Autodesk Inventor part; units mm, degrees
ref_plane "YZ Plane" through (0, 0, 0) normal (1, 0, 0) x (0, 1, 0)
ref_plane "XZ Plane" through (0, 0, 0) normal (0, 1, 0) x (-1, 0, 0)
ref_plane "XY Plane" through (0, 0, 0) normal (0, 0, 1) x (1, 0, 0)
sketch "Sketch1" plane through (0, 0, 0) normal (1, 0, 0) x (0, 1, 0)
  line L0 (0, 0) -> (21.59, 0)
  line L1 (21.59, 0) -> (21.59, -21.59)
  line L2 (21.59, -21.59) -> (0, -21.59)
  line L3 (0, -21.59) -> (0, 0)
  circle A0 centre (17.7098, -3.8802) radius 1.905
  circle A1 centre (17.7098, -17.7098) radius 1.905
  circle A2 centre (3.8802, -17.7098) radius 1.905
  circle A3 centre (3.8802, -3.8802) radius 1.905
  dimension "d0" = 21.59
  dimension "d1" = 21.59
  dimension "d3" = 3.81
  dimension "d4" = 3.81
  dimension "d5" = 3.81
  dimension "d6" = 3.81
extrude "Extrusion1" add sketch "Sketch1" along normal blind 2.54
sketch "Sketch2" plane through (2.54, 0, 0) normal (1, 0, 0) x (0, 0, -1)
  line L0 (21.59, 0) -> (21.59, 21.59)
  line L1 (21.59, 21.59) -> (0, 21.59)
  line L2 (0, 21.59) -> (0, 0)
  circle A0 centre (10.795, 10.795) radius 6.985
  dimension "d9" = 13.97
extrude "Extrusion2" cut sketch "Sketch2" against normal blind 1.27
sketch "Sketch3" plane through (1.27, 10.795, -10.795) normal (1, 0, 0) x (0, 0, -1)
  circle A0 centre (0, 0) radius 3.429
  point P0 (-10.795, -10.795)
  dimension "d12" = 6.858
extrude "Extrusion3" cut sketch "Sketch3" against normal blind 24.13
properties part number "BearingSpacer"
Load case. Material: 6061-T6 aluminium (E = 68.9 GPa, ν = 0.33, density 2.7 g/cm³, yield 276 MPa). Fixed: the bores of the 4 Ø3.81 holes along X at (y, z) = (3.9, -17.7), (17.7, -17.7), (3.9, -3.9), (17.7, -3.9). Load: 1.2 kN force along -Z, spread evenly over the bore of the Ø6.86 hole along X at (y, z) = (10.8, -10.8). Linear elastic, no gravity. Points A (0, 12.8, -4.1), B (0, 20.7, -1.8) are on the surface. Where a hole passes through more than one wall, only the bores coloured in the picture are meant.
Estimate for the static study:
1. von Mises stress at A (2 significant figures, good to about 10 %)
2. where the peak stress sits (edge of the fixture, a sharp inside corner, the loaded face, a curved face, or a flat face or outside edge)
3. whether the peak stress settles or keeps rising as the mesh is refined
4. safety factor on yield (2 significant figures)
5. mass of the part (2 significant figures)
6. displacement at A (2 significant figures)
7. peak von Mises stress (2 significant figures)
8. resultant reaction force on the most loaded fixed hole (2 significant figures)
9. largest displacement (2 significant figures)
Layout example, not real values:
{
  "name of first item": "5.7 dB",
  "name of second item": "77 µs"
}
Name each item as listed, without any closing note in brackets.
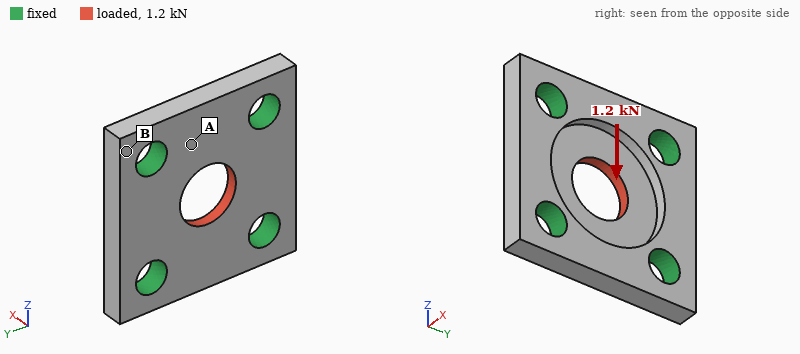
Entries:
{
  "von Mises stress at A": "26 MPa",
  "where the peak stress sits": "the loaded face",
  "whether the peak stress settles or keeps rising as the mesh is refined": "settles",
  "safety factor on yield": "3.6",
  "mass of the part": "2.2 g",
  "displacement at A": "2.6 µm",
  "peak von Mises stress": "77 MPa",
  "resultant reaction force on the most loaded fixed hole": "320 N",
  "largest displacement": "4.8 µm"
}
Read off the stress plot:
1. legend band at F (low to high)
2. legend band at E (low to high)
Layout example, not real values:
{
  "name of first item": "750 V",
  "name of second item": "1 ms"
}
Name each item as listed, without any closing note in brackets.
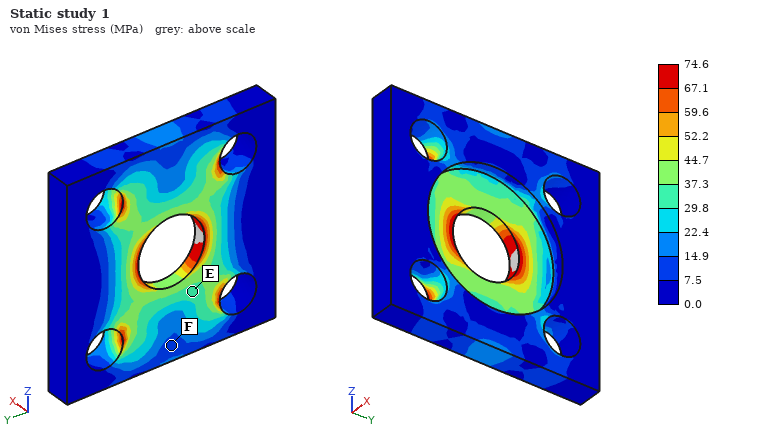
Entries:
{
  "legend band at F": "7.5 to 14.9 MPa",
  "legend band at E": "29.8 to 37.3 MPa"
}
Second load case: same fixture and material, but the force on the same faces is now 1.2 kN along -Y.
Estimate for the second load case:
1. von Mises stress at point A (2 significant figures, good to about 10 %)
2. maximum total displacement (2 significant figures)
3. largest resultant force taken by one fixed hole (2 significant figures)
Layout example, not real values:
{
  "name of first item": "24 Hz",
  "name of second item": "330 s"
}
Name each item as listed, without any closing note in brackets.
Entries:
{
  "von Mises stress at point A": "14 MPa",
  "maximum total displacement": "4.8 µm",
  "largest resultant force taken by one fixed hole": "320 N"
}
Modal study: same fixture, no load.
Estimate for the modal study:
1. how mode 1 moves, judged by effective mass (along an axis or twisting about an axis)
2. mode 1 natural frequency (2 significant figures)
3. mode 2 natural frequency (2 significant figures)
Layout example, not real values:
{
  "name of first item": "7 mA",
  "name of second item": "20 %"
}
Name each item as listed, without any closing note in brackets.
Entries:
{
  "how mode 1 moves, judged by effective mass": "along X",
  "mode 1 natural frequency": "65 kHz",
  "mode 2 natural frequency": "77 kHz"
}
